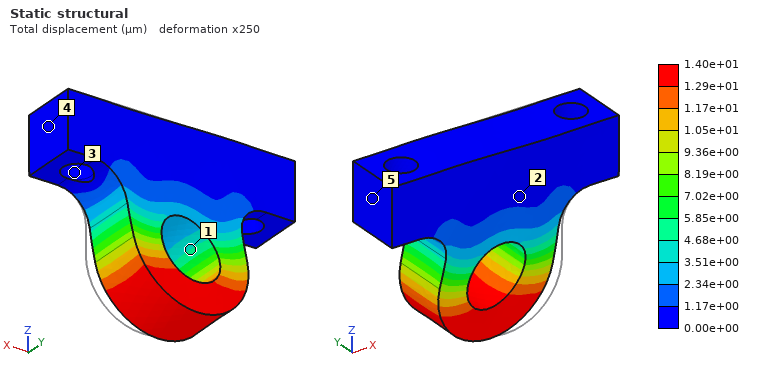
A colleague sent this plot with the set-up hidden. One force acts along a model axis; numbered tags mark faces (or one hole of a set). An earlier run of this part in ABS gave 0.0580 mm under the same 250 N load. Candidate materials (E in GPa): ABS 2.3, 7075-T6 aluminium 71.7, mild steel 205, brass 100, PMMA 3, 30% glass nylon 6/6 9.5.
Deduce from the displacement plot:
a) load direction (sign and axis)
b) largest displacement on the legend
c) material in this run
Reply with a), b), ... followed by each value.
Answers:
a) -X
b) 1.40e+01 µm
c) 30% glass nylon 6/6
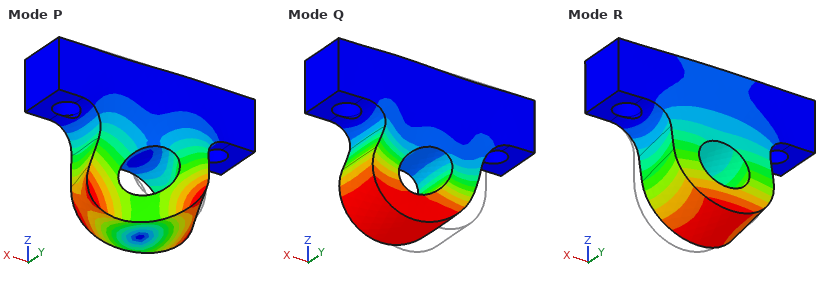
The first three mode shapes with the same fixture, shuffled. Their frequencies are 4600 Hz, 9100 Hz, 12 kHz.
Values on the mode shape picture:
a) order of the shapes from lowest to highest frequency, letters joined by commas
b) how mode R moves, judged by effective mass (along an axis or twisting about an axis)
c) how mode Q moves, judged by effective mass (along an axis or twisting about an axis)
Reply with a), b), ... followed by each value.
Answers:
a) R, Q, P
b) along Y
c) along X
